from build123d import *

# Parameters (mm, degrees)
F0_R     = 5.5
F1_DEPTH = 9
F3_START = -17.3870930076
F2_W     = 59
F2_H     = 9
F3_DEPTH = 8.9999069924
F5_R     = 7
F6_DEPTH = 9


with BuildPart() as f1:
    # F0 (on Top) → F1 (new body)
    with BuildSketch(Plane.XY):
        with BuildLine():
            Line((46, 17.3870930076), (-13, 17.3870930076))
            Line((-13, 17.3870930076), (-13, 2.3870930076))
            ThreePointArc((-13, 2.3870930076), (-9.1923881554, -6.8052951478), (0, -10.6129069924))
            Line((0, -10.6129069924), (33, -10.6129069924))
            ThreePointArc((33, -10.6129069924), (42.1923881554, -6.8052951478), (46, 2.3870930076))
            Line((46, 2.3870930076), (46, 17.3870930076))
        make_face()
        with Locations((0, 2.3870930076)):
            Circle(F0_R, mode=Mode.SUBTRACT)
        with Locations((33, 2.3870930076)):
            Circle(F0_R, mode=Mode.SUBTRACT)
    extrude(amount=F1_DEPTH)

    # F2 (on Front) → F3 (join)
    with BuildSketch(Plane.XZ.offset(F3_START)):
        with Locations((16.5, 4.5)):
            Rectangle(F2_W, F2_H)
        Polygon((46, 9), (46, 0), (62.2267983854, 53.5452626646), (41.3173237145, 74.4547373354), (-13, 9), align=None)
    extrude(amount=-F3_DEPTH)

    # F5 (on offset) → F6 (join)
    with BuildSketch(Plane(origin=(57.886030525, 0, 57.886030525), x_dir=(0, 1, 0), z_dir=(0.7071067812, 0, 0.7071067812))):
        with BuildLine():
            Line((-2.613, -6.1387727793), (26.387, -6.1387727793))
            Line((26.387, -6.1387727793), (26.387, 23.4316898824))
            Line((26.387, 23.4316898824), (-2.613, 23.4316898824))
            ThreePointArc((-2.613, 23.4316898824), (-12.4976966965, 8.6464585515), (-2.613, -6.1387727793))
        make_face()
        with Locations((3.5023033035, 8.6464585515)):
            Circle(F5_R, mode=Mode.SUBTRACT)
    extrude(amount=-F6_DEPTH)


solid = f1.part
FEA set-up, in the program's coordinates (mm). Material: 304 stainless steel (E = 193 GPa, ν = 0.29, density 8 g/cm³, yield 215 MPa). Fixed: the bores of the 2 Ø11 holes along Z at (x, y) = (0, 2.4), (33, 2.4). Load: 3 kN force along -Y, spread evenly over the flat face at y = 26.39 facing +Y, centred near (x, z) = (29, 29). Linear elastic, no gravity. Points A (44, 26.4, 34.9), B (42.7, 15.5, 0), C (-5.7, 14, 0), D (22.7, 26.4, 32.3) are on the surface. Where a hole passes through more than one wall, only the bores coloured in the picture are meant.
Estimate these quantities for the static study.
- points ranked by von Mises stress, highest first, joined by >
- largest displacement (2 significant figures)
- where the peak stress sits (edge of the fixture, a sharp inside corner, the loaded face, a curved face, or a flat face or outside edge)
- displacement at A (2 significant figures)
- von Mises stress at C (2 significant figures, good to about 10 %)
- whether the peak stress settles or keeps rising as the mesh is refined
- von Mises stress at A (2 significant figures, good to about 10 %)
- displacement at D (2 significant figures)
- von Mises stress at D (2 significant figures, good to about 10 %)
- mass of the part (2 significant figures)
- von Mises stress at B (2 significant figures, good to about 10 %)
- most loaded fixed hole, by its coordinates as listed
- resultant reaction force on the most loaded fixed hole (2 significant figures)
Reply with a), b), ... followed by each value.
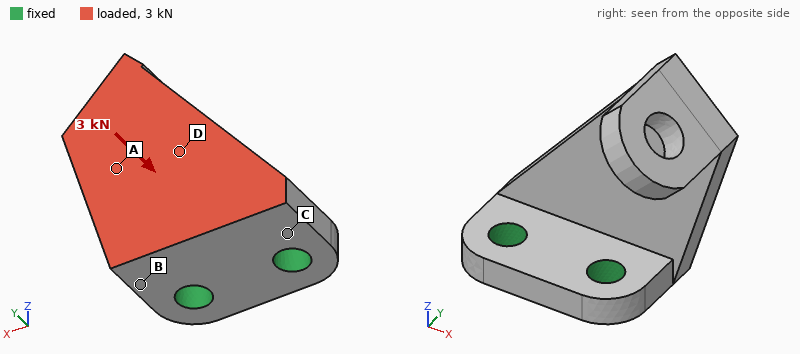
a) B > C > D > A
b) 0.27 mm
c) edge of the fixture
d) 0.10 mm
e) 61 MPa
f) keeps rising
g) 27 MPa
h) 0.080 mm
i) 43 MPa
j) 380 g
k) 96 MPa
l) (33, 2.4)
m) 2.5 kN
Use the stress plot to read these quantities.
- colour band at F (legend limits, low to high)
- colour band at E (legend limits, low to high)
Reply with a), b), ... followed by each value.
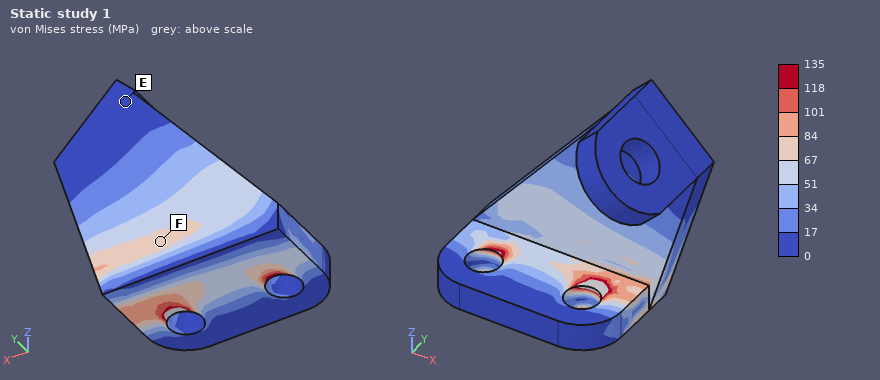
a) 67 to 84 MPa
b) 0 to 17 MPa
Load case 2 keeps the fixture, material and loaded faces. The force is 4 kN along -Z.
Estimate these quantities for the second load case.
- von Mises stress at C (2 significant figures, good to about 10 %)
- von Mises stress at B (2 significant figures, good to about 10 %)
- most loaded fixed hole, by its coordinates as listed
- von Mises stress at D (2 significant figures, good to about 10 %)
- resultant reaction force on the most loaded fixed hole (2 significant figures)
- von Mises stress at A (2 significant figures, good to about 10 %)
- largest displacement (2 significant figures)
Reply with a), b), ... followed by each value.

a) 47 MPa
b) 54 MPa
c) (33, 2.4)
d) 17 MPa
e) 3.2 kN
f) 16 MPa
g) 0.14 mm
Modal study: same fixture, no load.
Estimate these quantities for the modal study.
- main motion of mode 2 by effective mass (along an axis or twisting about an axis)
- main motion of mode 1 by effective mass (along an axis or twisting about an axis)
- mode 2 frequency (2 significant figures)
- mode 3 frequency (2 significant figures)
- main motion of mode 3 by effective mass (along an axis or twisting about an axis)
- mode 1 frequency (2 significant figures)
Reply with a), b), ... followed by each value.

a) along X
b) along Y
c) 2400 Hz
d) 3600 Hz
e) along Z
f) 1100 Hz
